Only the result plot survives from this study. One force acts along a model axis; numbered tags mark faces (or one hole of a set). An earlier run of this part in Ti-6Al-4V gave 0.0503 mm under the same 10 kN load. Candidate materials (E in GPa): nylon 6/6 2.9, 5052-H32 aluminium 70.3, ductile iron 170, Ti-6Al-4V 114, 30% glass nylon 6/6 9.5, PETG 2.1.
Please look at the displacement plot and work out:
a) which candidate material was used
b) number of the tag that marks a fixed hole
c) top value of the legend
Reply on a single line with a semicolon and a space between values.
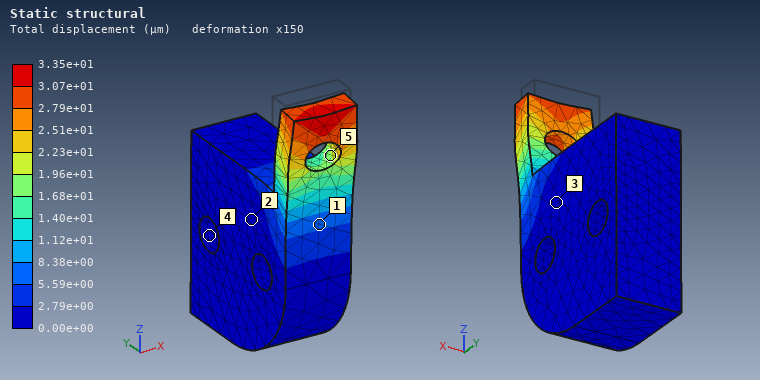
ductile iron; 4; 3.35e+01 µm
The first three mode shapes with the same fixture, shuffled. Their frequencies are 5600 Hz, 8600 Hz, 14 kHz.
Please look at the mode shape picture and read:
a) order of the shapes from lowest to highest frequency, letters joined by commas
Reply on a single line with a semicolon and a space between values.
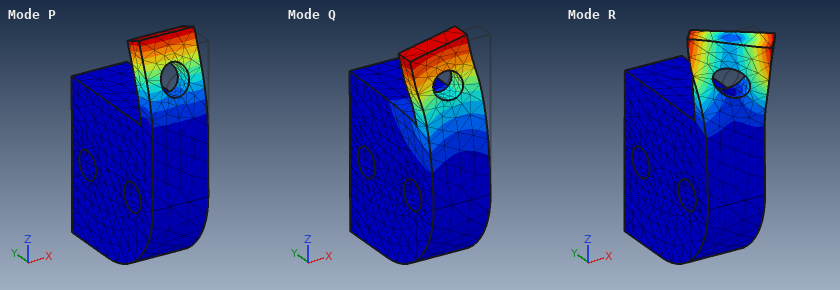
P, Q, R
